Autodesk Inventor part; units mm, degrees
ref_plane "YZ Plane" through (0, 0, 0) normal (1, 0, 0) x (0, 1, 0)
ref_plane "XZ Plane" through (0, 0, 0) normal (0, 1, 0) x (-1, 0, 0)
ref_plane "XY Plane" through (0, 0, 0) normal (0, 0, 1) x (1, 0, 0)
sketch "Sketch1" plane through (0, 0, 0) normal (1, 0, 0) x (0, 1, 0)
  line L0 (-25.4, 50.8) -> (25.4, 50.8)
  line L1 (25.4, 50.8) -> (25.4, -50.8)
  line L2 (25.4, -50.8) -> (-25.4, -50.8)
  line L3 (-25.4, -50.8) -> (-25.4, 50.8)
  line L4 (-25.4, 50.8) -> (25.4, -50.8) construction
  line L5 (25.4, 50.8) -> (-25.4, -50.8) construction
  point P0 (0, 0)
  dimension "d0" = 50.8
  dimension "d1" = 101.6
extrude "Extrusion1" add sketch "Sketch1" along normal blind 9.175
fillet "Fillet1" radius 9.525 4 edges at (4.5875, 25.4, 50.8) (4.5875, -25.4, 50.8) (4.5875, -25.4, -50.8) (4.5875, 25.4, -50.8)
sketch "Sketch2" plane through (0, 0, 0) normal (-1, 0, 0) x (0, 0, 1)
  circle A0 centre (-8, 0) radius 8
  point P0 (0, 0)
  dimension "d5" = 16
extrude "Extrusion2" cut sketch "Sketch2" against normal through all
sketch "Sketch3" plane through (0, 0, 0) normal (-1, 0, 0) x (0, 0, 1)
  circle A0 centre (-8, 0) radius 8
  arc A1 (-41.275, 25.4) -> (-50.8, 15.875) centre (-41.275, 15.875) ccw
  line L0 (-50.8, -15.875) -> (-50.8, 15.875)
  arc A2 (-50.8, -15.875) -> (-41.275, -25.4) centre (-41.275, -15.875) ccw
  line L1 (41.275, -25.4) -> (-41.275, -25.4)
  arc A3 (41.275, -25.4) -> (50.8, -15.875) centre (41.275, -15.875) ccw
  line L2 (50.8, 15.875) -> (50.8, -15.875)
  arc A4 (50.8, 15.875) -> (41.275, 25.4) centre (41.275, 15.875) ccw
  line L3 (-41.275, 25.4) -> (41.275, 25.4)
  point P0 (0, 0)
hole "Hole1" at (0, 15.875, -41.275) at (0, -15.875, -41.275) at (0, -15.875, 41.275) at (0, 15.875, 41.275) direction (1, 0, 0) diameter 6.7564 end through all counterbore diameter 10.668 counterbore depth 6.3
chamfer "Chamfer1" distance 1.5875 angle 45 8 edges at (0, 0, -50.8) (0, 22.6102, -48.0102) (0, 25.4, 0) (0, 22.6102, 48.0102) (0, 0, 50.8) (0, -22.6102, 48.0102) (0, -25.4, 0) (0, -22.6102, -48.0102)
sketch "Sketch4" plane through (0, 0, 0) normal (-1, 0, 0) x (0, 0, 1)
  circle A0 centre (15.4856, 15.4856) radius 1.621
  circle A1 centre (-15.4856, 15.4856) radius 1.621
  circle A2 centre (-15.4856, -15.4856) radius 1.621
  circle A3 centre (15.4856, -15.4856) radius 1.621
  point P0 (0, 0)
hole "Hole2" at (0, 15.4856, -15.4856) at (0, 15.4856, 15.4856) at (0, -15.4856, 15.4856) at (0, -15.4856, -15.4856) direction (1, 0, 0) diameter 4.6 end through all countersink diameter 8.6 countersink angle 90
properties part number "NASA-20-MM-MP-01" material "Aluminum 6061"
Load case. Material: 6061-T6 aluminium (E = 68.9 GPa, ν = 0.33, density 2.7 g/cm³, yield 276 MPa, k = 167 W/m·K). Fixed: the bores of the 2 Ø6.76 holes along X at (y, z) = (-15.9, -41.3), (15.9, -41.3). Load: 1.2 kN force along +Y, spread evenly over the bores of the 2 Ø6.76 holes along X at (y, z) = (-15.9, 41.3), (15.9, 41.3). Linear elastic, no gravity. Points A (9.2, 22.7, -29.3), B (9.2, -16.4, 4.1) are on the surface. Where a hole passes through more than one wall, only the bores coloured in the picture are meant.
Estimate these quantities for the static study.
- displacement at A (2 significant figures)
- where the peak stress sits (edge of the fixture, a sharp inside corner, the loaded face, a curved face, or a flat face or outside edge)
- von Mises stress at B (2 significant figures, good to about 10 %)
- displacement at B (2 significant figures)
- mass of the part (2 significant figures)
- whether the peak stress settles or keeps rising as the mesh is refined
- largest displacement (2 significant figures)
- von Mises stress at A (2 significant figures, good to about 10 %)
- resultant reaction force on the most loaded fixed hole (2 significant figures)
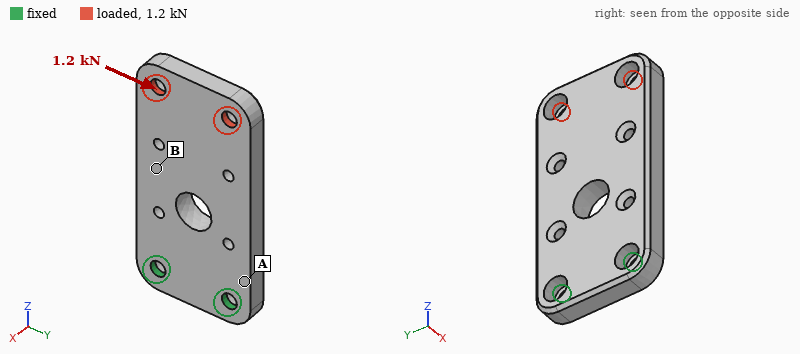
0.016 mm
edge of the fixture
13 MPa
0.049 mm
110 g
keeps rising
0.10 mm
29 MPa
2.8 kN
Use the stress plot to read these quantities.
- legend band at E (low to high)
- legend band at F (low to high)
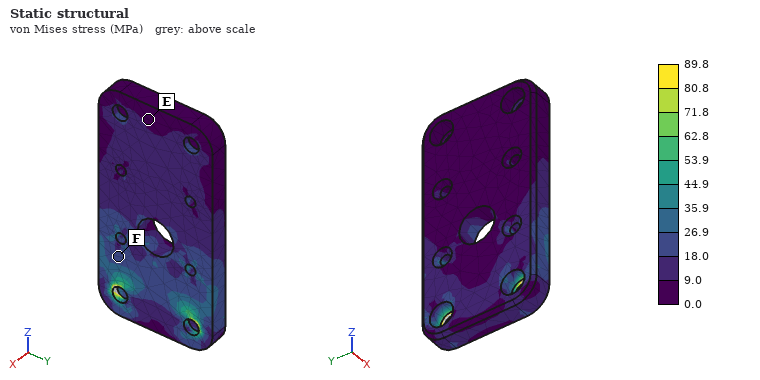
0.0 to 9.0 MPa
18.0 to 26.9 MPa
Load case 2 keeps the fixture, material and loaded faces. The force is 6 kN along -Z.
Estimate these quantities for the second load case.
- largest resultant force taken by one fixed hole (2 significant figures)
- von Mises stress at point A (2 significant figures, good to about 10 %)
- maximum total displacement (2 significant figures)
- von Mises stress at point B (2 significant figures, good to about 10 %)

3.0 kN
45 MPa
0.39 mm
46 MPa
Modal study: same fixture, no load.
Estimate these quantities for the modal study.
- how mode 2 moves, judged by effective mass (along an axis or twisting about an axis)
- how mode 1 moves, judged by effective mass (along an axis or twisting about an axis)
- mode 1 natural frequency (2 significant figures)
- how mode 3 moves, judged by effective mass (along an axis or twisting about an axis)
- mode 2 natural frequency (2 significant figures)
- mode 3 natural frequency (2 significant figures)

along Y
along X
630 Hz
along Y
2800 Hz
3400 Hz
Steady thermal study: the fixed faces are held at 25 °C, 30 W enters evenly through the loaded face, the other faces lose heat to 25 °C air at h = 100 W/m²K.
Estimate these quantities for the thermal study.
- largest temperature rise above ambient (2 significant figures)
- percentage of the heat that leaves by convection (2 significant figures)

29 K
54 %
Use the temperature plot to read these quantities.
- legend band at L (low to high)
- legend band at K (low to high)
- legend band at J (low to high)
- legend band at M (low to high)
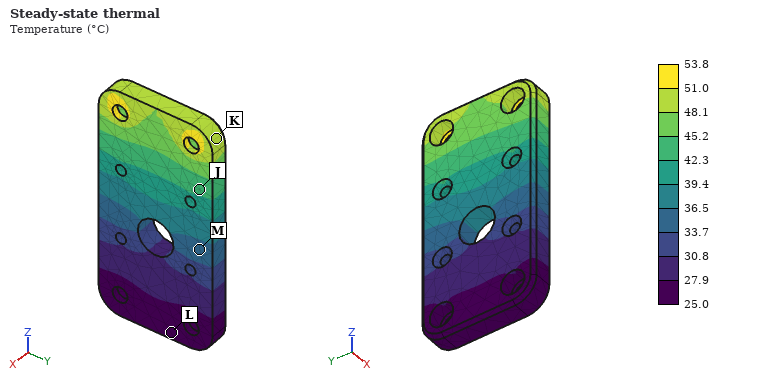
25.0 to 27.9 °C
48.1 to 51.0 °C
42.3 to 45.2 °C
33.7 to 36.5 °C
